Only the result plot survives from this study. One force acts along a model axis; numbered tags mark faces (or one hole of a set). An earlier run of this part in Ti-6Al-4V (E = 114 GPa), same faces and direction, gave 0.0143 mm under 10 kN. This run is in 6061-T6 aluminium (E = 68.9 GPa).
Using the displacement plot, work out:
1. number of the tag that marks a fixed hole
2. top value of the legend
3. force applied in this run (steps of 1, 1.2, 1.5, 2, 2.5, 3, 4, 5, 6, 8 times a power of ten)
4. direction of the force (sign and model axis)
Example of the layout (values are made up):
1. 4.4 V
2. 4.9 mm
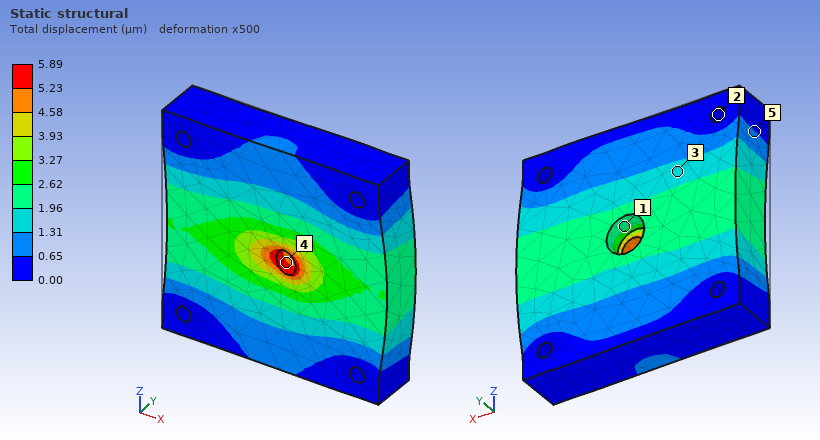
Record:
1. 2
2. 5.89 µm
3. 2.5 kN
4. +X
